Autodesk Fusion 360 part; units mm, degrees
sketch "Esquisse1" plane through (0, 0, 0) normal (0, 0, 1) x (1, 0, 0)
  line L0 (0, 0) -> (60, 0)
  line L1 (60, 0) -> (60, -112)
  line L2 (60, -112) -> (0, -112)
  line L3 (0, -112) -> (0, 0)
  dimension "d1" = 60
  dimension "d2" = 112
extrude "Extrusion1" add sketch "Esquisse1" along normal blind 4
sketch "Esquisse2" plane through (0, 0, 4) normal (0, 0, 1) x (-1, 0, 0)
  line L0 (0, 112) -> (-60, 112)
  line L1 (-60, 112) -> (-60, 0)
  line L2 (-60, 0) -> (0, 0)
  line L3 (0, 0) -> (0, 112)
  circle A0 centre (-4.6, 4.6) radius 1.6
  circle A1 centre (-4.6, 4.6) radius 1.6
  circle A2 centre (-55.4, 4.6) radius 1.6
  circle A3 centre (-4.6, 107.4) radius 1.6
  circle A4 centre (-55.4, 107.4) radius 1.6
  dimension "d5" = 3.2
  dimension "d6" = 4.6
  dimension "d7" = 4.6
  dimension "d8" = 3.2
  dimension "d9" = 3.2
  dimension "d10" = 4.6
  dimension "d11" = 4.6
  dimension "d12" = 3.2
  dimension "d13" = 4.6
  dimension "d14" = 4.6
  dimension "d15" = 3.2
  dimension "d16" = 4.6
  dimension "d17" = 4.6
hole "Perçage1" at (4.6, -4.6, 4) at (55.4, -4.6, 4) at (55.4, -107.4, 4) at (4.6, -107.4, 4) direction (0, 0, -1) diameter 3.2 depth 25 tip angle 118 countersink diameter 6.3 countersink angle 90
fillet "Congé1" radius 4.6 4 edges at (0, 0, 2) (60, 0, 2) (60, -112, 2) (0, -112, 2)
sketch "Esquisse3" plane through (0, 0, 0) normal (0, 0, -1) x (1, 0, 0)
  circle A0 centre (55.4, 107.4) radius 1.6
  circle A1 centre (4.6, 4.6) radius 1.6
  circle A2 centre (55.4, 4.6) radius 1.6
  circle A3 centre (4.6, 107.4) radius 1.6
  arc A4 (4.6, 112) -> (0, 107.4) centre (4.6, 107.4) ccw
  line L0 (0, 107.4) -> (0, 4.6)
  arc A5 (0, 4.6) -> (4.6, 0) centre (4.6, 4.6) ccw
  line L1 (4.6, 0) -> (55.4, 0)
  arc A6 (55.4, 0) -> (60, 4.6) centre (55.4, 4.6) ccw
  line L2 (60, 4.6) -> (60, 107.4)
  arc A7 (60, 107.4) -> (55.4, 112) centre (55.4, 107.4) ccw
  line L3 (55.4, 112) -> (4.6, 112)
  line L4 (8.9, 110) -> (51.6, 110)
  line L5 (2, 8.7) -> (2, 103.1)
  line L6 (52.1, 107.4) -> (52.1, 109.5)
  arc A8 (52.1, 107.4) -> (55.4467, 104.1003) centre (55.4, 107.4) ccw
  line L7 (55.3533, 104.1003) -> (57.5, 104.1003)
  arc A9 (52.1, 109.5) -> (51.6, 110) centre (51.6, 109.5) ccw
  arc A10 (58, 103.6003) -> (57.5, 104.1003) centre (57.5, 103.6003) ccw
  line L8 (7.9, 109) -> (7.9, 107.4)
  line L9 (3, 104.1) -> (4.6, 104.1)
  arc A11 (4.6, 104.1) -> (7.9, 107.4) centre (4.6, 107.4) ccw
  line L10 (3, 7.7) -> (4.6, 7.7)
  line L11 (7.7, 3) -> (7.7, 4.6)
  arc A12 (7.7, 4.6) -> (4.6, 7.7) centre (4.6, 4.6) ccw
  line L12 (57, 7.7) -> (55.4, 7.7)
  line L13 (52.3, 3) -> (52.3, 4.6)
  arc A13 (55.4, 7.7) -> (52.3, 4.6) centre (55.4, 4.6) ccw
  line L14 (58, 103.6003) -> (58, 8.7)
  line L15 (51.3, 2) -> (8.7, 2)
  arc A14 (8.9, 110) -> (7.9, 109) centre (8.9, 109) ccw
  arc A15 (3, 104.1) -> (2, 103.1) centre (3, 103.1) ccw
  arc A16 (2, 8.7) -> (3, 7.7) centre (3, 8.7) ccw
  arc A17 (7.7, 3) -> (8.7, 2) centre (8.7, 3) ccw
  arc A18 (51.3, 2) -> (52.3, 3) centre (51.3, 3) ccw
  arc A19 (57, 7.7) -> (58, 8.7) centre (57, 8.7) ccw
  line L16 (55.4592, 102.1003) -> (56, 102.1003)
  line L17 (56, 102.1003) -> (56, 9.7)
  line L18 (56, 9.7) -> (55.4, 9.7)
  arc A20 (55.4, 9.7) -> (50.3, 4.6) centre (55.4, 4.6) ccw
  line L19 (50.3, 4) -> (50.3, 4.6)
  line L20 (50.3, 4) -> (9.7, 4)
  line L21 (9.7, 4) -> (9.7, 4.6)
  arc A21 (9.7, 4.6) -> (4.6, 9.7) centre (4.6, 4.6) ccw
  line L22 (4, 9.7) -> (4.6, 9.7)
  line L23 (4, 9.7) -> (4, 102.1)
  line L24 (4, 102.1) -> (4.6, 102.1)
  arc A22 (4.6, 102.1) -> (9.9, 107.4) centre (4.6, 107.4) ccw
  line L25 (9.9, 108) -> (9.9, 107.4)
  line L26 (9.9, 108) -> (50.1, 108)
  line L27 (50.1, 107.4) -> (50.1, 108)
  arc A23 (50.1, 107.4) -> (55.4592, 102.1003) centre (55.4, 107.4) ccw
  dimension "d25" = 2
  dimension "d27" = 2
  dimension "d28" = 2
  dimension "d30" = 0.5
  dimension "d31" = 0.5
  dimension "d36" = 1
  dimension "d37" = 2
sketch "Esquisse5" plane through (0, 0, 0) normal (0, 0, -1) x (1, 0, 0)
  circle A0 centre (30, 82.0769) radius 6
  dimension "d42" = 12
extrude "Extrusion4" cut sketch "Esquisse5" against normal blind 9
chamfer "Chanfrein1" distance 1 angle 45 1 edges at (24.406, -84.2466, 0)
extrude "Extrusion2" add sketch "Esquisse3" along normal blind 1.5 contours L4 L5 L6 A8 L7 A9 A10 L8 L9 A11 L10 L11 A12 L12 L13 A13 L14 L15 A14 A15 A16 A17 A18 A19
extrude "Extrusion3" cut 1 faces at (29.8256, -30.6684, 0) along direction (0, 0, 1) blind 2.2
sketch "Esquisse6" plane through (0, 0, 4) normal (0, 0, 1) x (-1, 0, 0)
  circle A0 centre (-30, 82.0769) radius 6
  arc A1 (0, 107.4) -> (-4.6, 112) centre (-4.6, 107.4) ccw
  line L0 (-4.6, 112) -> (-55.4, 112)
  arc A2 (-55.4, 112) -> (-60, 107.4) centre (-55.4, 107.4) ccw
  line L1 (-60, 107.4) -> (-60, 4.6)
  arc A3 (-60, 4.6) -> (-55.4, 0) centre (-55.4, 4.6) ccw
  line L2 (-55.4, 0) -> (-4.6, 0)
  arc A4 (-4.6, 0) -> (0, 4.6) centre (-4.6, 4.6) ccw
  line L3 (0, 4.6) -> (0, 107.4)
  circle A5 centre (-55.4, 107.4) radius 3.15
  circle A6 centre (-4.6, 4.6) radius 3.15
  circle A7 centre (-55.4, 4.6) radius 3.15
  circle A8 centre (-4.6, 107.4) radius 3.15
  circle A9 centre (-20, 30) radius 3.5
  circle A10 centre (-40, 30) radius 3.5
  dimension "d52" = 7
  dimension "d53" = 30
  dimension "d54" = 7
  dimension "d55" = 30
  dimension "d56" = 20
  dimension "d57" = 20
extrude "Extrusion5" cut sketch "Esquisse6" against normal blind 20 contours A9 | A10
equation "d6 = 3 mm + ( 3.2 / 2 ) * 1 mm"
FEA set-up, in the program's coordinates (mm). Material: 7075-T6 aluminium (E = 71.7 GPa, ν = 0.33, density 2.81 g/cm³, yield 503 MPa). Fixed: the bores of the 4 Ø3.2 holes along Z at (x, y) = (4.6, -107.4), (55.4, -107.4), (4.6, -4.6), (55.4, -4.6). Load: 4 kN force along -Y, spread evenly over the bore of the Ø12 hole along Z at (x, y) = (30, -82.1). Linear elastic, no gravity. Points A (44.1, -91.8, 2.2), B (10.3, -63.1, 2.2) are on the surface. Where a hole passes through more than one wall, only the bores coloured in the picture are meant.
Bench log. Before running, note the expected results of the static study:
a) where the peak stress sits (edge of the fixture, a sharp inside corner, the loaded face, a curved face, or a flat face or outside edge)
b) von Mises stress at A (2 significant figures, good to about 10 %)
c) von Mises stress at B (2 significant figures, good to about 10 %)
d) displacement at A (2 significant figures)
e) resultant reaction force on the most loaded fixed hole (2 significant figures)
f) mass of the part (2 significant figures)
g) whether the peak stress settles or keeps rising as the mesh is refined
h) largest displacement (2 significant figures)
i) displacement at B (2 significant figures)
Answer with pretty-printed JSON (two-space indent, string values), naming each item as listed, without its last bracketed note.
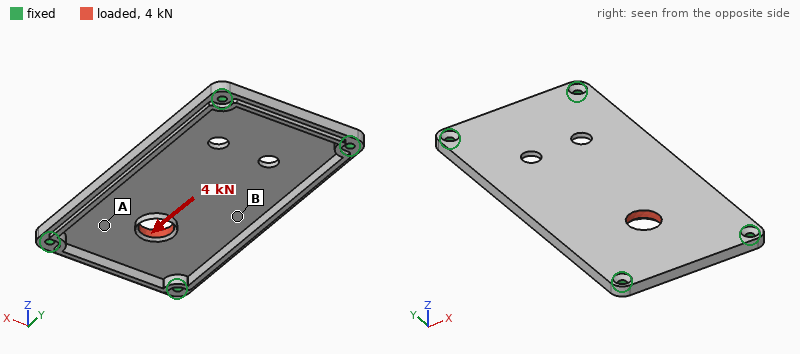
{
  "where the peak stress sits": "edge of the fixture",
  "von Mises stress at A": "48 MPa",
  "von Mises stress at B": "20 MPa",
  "displacement at A": "24 µm",
  "resultant reaction force on the most loaded fixed hole": "1.4 kN",
  "mass of the part": "44 g",
  "whether the peak stress settles or keeps rising as the mesh is refined": "keeps rising",
  "largest displacement": "65 µm",
  "displacement at B": "31 µm"
}
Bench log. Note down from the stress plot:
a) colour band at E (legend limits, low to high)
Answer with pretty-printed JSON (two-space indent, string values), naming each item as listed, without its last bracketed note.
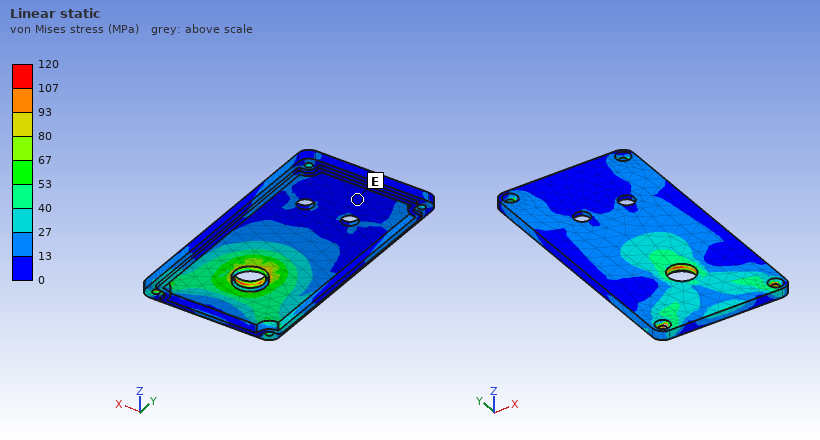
{
  "colour band at E": "0 to 13 MPa"
}
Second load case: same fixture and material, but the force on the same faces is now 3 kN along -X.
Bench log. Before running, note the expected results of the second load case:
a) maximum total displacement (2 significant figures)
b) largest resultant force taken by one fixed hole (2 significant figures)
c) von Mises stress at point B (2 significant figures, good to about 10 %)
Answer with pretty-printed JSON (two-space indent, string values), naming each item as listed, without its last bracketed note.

{
  "maximum total displacement": "71 µm",
  "largest resultant force taken by one fixed hole": "1.3 kN",
  "von Mises stress at point B": "15 MPa"
}
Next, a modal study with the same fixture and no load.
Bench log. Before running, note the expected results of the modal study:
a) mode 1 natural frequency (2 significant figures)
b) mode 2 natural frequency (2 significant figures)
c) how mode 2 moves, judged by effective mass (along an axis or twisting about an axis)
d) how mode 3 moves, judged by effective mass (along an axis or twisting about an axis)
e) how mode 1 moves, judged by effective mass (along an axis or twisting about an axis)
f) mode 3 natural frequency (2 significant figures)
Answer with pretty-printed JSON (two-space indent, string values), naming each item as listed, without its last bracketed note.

{
  "mode 1 natural frequency": "1500 Hz",
  "mode 2 natural frequency": "2200 Hz",
  "how mode 2 moves, judged by effective mass": "twisting about Y",
  "how mode 3 moves, judged by effective mass": "twisting about X",
  "how mode 1 moves, judged by effective mass": "along Z",
  "mode 3 natural frequency": "3400 Hz"
}
